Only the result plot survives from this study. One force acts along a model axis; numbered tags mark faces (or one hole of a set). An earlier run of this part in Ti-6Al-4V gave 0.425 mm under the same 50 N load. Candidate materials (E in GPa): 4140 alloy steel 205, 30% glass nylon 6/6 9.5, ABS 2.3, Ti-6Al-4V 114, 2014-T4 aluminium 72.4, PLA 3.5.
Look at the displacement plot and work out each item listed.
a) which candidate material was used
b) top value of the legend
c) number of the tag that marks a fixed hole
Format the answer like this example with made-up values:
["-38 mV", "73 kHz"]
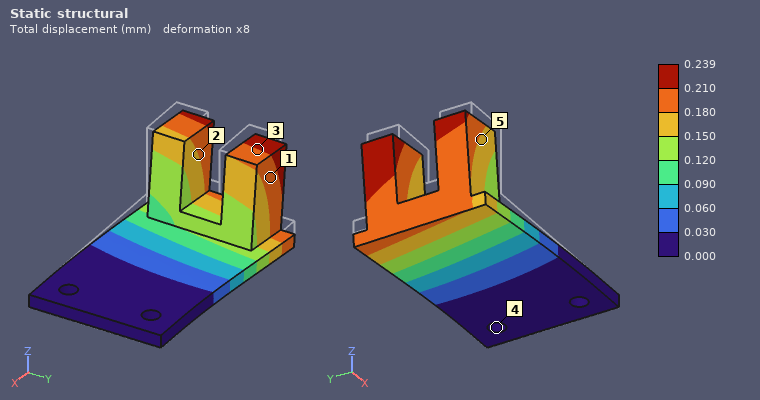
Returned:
["4140 alloy steel", "0.239 mm", "4"]
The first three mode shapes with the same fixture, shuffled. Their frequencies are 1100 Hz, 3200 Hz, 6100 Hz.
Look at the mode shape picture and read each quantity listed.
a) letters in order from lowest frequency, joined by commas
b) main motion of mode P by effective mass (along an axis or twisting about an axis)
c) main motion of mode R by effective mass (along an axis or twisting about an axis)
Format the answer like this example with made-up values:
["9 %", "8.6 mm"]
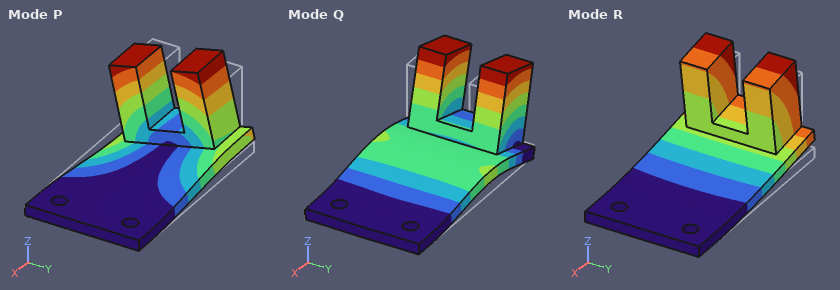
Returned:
["R, P, Q", "along Y", "along Z"]
